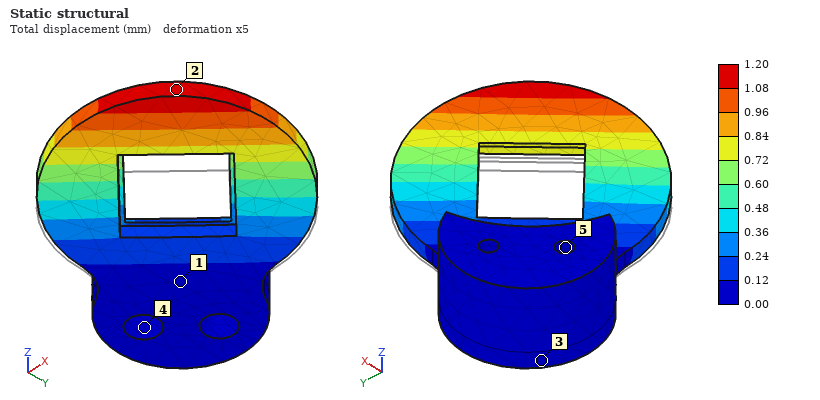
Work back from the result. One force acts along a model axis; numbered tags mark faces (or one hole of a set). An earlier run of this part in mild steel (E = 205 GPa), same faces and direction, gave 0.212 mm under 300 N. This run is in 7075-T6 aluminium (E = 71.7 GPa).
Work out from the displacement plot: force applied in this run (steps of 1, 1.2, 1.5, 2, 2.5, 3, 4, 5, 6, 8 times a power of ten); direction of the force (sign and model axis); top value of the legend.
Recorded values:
600 N
+Z
1.20 mm
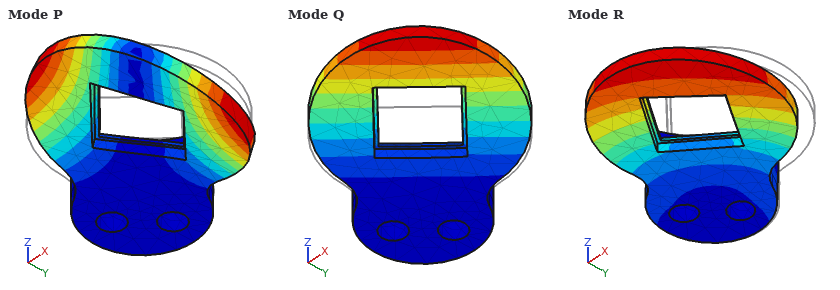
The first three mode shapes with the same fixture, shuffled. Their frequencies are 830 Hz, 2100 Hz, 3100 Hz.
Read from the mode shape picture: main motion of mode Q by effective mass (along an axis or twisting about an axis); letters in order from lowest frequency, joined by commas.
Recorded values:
along Z
Q, P, R
